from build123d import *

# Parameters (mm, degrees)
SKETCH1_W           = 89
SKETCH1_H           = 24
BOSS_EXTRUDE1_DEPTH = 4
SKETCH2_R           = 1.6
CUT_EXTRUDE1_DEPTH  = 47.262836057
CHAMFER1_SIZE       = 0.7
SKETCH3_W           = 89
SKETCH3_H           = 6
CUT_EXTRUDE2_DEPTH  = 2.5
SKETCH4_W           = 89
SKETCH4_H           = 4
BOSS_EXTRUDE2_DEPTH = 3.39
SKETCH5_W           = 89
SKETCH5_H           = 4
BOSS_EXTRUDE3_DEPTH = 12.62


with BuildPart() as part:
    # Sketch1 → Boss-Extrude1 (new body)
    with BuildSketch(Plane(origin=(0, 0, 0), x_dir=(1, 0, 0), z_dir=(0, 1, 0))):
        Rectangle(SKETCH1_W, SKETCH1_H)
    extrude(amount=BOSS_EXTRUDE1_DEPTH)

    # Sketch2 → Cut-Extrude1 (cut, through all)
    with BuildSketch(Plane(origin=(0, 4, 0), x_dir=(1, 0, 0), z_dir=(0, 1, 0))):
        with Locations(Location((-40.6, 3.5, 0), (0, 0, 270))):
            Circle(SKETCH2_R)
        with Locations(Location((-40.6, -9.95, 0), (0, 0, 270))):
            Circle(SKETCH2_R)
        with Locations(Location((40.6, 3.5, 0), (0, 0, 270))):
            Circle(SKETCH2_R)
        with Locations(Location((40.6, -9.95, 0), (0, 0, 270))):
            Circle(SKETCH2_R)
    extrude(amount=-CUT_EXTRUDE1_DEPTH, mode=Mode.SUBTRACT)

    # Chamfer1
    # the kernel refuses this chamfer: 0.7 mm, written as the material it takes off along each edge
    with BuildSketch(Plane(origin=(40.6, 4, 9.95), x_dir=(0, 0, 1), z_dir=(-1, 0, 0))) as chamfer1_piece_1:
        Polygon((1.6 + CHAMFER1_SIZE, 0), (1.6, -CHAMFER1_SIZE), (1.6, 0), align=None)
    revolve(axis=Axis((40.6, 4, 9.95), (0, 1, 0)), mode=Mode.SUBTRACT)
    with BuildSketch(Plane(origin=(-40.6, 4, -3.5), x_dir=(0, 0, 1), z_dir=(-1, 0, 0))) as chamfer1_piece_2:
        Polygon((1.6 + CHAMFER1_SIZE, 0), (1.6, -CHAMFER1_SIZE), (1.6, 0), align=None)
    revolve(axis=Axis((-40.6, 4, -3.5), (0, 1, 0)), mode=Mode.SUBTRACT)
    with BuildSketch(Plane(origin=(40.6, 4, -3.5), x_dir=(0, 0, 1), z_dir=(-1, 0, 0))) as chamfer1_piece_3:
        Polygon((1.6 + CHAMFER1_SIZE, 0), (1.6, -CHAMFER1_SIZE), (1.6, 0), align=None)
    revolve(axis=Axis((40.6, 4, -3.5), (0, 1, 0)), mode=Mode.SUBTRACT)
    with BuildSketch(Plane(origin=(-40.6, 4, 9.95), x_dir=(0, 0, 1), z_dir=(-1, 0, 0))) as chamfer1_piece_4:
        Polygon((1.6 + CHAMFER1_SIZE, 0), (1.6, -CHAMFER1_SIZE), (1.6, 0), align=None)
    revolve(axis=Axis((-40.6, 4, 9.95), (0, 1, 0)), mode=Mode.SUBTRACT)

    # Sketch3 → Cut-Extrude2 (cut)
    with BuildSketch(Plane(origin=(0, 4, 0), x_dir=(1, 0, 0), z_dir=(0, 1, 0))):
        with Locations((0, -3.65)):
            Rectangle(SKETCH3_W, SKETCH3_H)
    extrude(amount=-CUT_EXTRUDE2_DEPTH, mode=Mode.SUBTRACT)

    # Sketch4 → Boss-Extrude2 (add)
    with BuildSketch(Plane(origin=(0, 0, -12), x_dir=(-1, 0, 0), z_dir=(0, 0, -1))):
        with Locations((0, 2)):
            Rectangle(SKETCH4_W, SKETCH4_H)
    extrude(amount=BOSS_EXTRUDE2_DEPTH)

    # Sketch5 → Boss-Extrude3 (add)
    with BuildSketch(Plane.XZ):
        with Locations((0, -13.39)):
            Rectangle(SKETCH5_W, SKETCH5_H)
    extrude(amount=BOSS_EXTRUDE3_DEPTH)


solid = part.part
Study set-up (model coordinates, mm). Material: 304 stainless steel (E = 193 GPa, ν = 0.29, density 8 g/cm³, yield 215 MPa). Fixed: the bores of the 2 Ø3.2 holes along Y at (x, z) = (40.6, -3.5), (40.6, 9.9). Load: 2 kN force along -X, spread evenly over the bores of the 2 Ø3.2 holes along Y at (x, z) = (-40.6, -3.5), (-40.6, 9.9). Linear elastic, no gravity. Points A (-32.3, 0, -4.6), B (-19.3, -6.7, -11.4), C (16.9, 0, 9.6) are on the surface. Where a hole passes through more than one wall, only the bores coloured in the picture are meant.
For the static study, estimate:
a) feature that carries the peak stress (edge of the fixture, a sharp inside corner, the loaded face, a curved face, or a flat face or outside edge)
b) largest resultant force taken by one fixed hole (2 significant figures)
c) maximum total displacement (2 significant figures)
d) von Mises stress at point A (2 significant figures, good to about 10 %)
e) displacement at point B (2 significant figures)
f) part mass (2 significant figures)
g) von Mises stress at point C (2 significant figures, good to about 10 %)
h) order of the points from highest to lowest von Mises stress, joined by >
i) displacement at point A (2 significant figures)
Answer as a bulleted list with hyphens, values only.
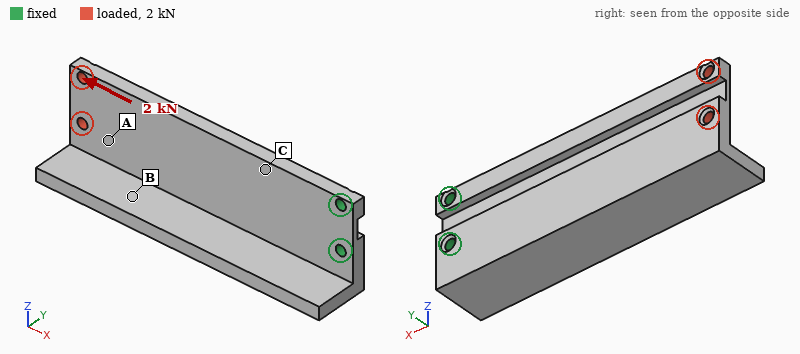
- the loaded face
- 1.0 kN
- 44 µm
- 21 MPa
- 17 µm
- 100 g
- 44 MPa
- C > A > B
- 26 µm
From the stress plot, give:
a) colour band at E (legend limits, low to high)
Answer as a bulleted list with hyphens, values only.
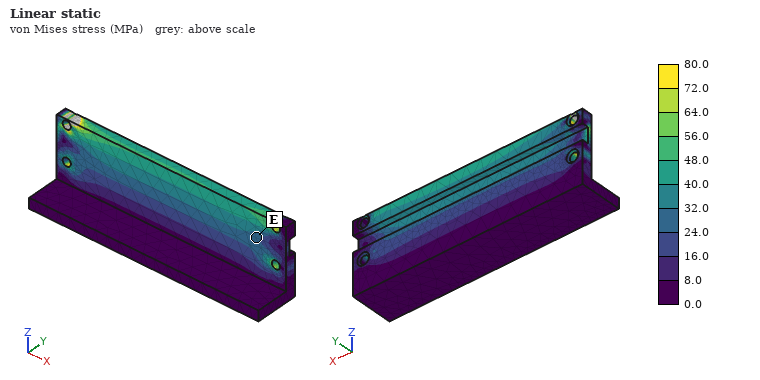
- 24.0 to 32.0 MPa
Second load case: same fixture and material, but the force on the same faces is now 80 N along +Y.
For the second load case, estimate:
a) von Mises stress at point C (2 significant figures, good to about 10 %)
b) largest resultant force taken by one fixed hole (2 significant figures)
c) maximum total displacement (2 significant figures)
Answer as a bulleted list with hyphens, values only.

- 20 MPa
- 110 N
- 0.26 mm
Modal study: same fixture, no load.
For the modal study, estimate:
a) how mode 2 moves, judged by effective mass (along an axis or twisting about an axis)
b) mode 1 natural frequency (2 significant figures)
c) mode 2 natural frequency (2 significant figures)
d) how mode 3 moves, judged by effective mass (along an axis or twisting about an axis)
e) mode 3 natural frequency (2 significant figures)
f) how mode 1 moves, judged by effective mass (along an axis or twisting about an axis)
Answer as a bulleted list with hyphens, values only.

- along Z
- 520 Hz
- 1800 Hz
- along Z
- 2000 Hz
- along Y
